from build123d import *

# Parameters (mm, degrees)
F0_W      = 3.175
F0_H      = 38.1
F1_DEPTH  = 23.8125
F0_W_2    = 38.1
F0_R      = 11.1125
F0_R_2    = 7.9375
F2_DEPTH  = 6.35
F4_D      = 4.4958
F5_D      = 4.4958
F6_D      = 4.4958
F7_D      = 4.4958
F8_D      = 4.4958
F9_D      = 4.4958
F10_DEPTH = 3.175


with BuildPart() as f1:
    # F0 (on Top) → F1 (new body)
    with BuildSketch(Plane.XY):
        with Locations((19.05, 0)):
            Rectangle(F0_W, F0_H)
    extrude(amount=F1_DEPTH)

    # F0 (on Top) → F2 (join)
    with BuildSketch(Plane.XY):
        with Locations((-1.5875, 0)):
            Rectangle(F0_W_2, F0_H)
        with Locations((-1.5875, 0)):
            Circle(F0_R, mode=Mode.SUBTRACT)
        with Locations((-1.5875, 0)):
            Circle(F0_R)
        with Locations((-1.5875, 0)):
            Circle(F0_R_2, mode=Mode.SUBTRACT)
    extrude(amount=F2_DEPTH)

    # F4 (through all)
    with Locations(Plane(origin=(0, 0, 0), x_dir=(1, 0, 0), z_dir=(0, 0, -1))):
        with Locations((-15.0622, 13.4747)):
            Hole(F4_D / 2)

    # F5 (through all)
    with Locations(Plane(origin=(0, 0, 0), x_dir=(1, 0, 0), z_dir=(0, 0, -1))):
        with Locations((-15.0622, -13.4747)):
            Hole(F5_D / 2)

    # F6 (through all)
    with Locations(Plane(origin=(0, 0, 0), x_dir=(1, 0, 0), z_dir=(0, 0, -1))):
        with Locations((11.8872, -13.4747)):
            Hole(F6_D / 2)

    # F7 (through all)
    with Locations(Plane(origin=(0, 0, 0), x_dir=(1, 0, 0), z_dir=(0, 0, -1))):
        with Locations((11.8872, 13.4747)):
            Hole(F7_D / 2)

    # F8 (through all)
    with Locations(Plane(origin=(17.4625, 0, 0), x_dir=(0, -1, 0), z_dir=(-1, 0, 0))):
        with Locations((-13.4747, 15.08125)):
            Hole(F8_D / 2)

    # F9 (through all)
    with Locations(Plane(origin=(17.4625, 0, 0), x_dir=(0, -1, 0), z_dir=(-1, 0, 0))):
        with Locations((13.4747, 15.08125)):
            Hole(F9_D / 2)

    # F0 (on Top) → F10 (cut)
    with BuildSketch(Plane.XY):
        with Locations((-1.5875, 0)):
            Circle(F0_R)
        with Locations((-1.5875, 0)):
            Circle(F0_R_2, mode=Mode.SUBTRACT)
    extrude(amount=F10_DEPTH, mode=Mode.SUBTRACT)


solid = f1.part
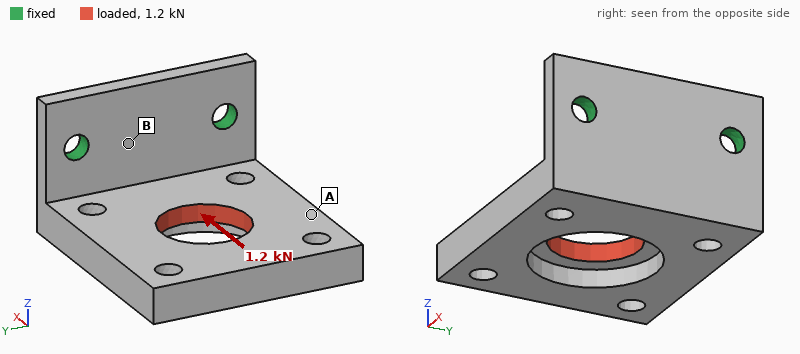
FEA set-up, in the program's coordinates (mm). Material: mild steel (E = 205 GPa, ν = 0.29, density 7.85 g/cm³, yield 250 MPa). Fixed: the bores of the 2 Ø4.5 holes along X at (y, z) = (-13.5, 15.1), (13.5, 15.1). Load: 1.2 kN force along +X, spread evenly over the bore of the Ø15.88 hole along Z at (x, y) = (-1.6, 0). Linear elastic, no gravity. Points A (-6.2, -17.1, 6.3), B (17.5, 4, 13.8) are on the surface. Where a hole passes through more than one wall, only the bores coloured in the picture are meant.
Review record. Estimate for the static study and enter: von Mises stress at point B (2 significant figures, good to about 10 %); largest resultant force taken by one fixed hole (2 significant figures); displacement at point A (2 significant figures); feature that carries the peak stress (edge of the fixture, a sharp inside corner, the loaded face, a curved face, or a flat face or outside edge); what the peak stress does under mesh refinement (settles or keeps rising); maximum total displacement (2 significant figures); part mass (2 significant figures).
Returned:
57 MPa
600 N
0.069 mm
edge of the fixture
keeps rising
0.11 mm
76 g
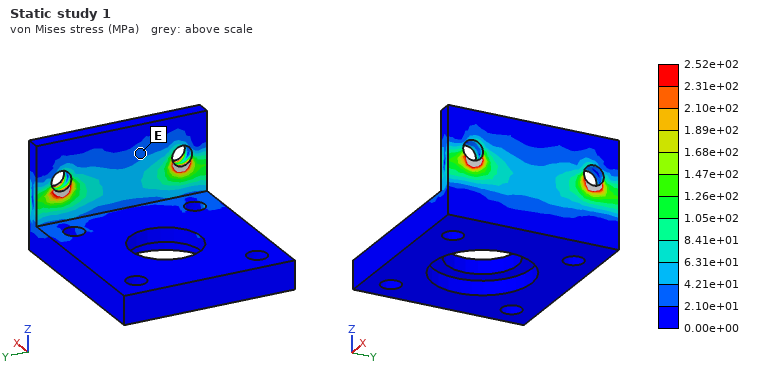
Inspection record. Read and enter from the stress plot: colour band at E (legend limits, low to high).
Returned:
2.10e+01 to 4.21e+01 MPa
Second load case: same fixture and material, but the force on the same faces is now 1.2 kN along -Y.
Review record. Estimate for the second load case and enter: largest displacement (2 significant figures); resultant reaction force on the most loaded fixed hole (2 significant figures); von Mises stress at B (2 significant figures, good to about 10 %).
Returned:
59 µm
1.1 kN
39 MPa
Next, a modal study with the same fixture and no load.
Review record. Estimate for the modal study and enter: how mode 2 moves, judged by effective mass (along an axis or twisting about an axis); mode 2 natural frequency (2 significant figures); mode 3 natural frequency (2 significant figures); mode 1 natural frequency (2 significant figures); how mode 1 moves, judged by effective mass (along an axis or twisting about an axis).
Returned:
along Y
3500 Hz
5700 Hz
1200 Hz
along Z
